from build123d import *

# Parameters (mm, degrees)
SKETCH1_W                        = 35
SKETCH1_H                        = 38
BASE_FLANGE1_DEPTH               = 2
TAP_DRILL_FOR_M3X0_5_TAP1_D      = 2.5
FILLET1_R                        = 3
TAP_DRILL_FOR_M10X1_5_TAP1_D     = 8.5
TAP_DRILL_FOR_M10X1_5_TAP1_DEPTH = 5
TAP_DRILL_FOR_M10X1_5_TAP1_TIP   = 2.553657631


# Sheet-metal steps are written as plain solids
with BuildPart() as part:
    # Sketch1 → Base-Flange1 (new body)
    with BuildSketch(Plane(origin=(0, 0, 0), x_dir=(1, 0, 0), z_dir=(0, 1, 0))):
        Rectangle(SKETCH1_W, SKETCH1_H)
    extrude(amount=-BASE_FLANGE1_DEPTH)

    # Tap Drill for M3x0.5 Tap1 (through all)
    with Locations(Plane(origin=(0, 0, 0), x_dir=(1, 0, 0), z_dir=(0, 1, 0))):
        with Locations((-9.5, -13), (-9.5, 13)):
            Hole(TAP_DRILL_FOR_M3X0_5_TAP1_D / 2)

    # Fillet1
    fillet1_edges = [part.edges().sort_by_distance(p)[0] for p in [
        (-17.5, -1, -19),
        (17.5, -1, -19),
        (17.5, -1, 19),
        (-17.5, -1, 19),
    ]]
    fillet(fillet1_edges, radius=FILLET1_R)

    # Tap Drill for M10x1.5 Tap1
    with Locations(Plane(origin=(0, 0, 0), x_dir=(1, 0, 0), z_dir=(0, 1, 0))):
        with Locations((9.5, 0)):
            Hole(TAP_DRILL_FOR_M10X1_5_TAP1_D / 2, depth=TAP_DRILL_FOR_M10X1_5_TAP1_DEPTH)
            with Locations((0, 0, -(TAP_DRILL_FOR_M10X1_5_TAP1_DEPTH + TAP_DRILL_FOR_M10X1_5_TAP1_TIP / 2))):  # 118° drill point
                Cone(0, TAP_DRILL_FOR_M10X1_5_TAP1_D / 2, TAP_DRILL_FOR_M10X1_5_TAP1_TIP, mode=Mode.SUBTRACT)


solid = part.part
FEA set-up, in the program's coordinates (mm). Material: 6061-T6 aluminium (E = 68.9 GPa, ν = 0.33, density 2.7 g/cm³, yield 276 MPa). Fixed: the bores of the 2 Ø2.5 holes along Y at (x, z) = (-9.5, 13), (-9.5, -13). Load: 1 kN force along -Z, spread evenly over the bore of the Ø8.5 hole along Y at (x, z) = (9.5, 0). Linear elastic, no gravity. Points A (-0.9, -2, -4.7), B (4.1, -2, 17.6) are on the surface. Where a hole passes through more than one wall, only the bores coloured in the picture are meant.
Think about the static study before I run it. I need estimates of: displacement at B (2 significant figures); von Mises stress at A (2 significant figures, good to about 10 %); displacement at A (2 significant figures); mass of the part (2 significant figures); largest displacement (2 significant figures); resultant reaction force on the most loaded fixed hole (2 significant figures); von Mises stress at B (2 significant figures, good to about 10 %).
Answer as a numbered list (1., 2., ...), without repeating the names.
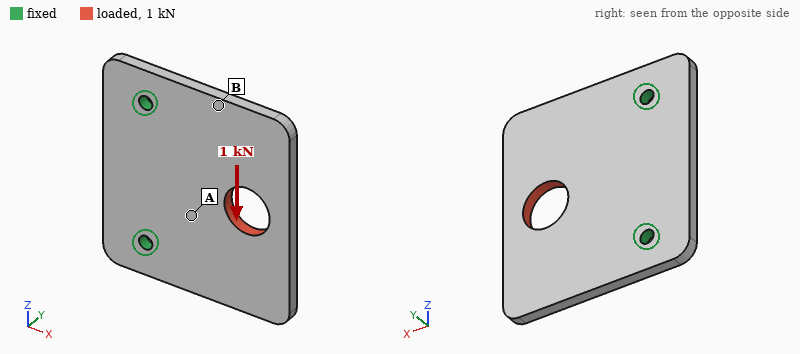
1. 15 µm
2. 34 MPa
3. 8.0 µm
4. 6.8 g
5. 27 µm
6. 860 N
7. 13 MPa
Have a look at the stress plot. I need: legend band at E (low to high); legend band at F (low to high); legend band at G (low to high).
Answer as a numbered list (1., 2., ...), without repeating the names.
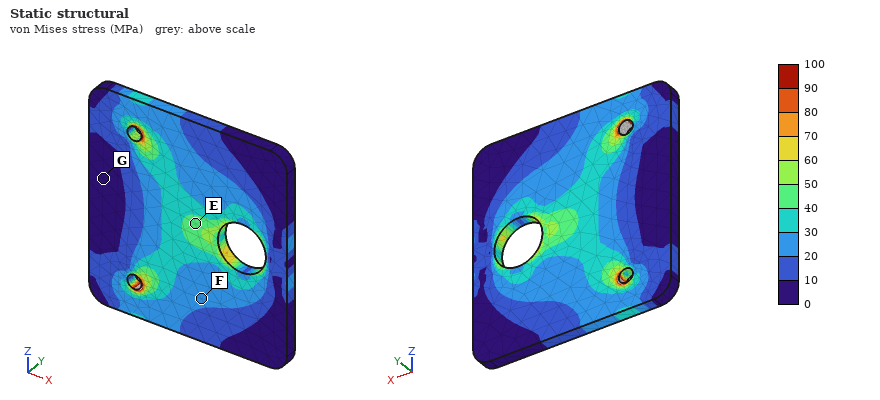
1. 40 to 50 MPa
2. 20 to 30 MPa
3. 0 to 10 MPa
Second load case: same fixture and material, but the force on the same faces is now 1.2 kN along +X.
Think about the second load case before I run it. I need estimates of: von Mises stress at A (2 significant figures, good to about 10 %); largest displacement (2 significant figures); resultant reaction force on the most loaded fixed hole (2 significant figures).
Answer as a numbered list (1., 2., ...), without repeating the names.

1. 21 MPa
2. 15 µm
3. 620 N
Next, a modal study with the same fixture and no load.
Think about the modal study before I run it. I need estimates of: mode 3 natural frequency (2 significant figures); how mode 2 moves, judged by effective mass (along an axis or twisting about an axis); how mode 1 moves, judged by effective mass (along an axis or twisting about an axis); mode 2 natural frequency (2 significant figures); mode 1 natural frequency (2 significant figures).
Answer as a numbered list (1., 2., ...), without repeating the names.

1. 9200 Hz
2. twisting about X
3. along Y
4. 4200 Hz
5. 2200 Hz
